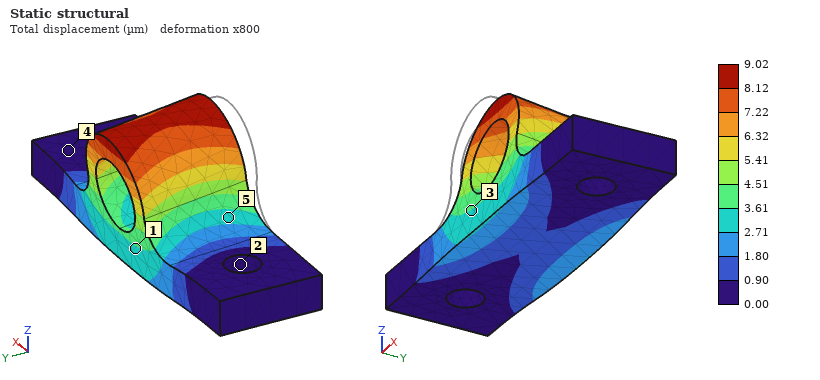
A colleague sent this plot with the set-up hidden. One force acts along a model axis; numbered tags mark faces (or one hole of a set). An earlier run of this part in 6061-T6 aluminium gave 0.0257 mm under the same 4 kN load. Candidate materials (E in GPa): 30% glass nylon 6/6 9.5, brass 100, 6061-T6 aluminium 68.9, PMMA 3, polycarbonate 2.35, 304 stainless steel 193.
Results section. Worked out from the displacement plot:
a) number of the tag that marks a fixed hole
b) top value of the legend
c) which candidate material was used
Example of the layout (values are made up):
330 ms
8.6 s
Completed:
2
9.02 µm
304 stainless steel
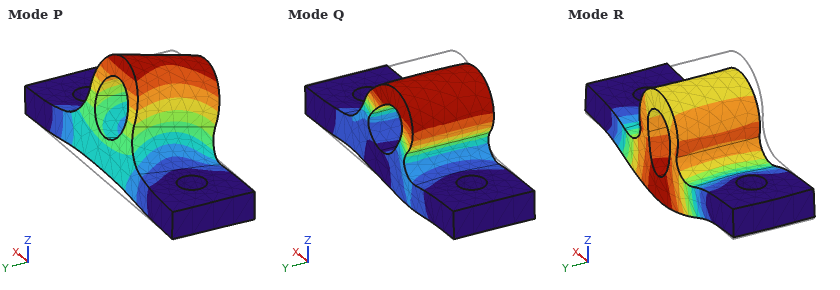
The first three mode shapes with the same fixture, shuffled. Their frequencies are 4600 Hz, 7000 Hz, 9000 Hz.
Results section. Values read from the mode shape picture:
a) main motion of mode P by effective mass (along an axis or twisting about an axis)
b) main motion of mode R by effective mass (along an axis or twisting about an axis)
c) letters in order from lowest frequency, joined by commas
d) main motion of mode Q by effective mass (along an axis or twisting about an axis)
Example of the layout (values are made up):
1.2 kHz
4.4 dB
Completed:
along Y
along Z
P, R, Q
along X
